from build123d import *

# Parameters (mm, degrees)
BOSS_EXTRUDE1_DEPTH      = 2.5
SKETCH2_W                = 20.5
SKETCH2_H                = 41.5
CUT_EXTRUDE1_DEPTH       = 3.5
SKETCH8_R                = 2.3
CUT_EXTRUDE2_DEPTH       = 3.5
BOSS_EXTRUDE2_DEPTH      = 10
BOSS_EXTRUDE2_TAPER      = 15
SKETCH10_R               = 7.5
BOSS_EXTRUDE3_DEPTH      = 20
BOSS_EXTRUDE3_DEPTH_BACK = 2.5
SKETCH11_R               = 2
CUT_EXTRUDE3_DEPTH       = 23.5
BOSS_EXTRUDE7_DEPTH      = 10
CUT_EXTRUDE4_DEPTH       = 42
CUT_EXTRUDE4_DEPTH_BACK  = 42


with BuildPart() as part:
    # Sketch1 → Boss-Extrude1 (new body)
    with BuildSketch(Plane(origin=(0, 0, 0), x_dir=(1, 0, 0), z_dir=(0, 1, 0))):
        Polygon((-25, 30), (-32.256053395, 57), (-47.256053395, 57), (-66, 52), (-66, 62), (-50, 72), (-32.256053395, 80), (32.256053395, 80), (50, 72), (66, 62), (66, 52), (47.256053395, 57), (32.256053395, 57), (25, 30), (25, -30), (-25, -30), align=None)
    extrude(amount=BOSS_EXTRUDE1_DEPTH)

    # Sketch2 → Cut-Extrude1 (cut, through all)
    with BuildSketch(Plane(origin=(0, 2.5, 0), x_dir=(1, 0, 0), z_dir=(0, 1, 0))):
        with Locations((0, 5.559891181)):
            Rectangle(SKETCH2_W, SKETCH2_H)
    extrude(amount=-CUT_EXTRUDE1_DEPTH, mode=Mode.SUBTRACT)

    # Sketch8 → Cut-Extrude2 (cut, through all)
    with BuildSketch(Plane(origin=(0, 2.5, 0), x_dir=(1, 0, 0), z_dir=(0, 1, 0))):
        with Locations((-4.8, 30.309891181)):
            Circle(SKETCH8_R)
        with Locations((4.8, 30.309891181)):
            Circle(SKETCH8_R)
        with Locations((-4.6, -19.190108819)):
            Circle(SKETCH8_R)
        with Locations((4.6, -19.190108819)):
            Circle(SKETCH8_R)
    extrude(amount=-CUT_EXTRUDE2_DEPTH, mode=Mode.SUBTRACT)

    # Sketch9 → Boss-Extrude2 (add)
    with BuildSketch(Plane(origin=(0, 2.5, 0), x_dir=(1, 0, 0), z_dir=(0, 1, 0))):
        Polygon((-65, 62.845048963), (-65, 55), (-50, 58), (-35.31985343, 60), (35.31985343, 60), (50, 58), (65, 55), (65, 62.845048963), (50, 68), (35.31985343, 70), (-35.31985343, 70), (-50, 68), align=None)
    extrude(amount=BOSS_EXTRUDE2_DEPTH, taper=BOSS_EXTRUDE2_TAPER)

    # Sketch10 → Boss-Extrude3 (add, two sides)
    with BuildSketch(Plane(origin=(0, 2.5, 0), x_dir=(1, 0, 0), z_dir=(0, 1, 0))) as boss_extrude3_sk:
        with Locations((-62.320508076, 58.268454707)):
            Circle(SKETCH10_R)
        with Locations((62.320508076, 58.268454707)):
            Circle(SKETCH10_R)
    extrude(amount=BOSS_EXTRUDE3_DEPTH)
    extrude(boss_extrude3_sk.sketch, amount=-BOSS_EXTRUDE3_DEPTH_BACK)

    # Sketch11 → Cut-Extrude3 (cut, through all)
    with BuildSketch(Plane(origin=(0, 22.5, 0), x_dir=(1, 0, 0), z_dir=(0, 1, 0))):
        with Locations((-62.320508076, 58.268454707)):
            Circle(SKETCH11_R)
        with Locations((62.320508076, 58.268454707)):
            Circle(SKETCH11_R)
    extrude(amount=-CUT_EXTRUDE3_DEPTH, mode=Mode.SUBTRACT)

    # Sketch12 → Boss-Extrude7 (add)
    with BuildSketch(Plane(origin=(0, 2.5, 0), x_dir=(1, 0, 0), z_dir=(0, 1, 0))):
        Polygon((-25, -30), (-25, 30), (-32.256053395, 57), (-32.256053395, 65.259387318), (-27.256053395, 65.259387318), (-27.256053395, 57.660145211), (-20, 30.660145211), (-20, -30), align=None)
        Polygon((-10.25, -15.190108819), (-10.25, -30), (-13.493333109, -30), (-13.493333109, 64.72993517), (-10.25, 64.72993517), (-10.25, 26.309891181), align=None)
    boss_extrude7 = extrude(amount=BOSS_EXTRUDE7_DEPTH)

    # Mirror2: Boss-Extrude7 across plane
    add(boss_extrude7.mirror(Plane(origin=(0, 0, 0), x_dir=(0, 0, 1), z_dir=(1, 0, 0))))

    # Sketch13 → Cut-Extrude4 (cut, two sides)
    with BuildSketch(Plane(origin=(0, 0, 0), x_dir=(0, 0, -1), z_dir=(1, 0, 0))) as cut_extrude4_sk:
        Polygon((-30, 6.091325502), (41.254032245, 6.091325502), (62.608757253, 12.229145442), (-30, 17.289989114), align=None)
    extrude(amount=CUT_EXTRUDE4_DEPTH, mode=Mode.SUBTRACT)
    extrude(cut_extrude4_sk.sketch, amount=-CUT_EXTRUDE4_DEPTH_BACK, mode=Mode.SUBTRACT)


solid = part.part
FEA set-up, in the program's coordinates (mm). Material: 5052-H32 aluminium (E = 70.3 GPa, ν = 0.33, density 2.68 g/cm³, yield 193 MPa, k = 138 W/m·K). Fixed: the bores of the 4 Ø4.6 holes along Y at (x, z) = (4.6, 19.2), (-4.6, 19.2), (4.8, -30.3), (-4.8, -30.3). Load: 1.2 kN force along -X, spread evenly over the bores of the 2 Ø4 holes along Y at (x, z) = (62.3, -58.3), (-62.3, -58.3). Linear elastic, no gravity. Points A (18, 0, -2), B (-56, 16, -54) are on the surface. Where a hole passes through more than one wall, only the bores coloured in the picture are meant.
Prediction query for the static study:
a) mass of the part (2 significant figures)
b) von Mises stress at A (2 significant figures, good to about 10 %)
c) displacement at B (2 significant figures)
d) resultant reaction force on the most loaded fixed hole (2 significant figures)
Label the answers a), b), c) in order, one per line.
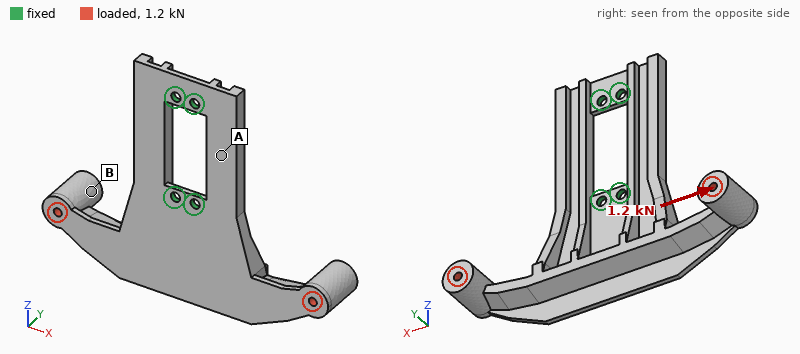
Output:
a) 99 g
b) 28 MPa
c) 0.74 mm
d) 1.4 kN
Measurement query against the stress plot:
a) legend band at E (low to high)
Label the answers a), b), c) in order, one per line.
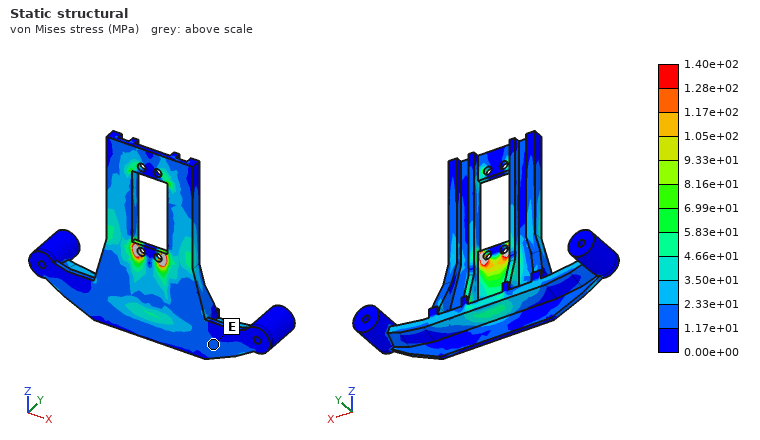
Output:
a) 1.17e+01 to 2.33e+01 MPa
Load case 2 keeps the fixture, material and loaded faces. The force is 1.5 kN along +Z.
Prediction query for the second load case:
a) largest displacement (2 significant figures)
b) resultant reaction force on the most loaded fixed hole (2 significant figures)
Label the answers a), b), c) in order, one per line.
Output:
a) 0.58 mm
b) 540 N
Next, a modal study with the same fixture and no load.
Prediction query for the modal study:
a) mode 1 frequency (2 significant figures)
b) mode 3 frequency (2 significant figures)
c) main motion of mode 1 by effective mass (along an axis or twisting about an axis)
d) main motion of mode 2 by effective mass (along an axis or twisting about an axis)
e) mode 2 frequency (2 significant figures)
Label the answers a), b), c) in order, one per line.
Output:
a) 450 Hz
b) 2100 Hz
c) twisting about Z
d) along Y
e) 720 Hz
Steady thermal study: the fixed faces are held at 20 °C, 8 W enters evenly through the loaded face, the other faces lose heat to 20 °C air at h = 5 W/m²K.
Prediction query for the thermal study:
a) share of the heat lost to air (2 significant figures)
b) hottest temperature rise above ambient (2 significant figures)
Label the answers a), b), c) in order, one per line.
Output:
a) 11 %
b) 20 K
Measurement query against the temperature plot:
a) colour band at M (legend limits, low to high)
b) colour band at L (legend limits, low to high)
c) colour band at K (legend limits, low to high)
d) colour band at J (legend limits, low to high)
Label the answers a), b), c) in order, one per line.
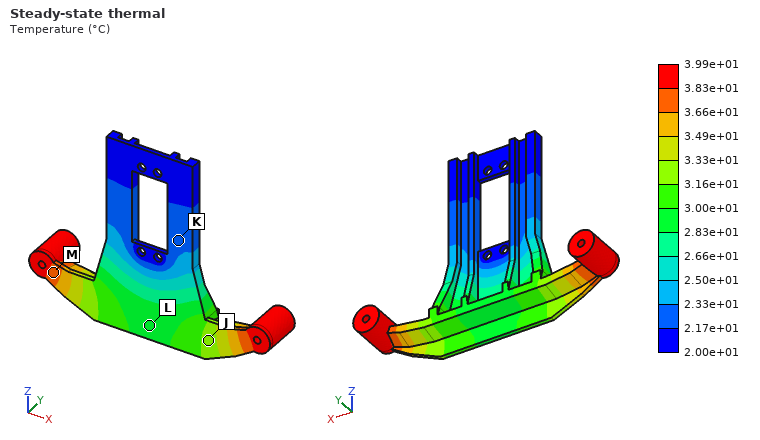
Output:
a) 3.66e+01 to 3.83e+01 °C
b) 2.83e+01 to 3.00e+01 °C
c) 2.17e+01 to 2.33e+01 °C
d) 3.16e+01 to 3.33e+01 °C
